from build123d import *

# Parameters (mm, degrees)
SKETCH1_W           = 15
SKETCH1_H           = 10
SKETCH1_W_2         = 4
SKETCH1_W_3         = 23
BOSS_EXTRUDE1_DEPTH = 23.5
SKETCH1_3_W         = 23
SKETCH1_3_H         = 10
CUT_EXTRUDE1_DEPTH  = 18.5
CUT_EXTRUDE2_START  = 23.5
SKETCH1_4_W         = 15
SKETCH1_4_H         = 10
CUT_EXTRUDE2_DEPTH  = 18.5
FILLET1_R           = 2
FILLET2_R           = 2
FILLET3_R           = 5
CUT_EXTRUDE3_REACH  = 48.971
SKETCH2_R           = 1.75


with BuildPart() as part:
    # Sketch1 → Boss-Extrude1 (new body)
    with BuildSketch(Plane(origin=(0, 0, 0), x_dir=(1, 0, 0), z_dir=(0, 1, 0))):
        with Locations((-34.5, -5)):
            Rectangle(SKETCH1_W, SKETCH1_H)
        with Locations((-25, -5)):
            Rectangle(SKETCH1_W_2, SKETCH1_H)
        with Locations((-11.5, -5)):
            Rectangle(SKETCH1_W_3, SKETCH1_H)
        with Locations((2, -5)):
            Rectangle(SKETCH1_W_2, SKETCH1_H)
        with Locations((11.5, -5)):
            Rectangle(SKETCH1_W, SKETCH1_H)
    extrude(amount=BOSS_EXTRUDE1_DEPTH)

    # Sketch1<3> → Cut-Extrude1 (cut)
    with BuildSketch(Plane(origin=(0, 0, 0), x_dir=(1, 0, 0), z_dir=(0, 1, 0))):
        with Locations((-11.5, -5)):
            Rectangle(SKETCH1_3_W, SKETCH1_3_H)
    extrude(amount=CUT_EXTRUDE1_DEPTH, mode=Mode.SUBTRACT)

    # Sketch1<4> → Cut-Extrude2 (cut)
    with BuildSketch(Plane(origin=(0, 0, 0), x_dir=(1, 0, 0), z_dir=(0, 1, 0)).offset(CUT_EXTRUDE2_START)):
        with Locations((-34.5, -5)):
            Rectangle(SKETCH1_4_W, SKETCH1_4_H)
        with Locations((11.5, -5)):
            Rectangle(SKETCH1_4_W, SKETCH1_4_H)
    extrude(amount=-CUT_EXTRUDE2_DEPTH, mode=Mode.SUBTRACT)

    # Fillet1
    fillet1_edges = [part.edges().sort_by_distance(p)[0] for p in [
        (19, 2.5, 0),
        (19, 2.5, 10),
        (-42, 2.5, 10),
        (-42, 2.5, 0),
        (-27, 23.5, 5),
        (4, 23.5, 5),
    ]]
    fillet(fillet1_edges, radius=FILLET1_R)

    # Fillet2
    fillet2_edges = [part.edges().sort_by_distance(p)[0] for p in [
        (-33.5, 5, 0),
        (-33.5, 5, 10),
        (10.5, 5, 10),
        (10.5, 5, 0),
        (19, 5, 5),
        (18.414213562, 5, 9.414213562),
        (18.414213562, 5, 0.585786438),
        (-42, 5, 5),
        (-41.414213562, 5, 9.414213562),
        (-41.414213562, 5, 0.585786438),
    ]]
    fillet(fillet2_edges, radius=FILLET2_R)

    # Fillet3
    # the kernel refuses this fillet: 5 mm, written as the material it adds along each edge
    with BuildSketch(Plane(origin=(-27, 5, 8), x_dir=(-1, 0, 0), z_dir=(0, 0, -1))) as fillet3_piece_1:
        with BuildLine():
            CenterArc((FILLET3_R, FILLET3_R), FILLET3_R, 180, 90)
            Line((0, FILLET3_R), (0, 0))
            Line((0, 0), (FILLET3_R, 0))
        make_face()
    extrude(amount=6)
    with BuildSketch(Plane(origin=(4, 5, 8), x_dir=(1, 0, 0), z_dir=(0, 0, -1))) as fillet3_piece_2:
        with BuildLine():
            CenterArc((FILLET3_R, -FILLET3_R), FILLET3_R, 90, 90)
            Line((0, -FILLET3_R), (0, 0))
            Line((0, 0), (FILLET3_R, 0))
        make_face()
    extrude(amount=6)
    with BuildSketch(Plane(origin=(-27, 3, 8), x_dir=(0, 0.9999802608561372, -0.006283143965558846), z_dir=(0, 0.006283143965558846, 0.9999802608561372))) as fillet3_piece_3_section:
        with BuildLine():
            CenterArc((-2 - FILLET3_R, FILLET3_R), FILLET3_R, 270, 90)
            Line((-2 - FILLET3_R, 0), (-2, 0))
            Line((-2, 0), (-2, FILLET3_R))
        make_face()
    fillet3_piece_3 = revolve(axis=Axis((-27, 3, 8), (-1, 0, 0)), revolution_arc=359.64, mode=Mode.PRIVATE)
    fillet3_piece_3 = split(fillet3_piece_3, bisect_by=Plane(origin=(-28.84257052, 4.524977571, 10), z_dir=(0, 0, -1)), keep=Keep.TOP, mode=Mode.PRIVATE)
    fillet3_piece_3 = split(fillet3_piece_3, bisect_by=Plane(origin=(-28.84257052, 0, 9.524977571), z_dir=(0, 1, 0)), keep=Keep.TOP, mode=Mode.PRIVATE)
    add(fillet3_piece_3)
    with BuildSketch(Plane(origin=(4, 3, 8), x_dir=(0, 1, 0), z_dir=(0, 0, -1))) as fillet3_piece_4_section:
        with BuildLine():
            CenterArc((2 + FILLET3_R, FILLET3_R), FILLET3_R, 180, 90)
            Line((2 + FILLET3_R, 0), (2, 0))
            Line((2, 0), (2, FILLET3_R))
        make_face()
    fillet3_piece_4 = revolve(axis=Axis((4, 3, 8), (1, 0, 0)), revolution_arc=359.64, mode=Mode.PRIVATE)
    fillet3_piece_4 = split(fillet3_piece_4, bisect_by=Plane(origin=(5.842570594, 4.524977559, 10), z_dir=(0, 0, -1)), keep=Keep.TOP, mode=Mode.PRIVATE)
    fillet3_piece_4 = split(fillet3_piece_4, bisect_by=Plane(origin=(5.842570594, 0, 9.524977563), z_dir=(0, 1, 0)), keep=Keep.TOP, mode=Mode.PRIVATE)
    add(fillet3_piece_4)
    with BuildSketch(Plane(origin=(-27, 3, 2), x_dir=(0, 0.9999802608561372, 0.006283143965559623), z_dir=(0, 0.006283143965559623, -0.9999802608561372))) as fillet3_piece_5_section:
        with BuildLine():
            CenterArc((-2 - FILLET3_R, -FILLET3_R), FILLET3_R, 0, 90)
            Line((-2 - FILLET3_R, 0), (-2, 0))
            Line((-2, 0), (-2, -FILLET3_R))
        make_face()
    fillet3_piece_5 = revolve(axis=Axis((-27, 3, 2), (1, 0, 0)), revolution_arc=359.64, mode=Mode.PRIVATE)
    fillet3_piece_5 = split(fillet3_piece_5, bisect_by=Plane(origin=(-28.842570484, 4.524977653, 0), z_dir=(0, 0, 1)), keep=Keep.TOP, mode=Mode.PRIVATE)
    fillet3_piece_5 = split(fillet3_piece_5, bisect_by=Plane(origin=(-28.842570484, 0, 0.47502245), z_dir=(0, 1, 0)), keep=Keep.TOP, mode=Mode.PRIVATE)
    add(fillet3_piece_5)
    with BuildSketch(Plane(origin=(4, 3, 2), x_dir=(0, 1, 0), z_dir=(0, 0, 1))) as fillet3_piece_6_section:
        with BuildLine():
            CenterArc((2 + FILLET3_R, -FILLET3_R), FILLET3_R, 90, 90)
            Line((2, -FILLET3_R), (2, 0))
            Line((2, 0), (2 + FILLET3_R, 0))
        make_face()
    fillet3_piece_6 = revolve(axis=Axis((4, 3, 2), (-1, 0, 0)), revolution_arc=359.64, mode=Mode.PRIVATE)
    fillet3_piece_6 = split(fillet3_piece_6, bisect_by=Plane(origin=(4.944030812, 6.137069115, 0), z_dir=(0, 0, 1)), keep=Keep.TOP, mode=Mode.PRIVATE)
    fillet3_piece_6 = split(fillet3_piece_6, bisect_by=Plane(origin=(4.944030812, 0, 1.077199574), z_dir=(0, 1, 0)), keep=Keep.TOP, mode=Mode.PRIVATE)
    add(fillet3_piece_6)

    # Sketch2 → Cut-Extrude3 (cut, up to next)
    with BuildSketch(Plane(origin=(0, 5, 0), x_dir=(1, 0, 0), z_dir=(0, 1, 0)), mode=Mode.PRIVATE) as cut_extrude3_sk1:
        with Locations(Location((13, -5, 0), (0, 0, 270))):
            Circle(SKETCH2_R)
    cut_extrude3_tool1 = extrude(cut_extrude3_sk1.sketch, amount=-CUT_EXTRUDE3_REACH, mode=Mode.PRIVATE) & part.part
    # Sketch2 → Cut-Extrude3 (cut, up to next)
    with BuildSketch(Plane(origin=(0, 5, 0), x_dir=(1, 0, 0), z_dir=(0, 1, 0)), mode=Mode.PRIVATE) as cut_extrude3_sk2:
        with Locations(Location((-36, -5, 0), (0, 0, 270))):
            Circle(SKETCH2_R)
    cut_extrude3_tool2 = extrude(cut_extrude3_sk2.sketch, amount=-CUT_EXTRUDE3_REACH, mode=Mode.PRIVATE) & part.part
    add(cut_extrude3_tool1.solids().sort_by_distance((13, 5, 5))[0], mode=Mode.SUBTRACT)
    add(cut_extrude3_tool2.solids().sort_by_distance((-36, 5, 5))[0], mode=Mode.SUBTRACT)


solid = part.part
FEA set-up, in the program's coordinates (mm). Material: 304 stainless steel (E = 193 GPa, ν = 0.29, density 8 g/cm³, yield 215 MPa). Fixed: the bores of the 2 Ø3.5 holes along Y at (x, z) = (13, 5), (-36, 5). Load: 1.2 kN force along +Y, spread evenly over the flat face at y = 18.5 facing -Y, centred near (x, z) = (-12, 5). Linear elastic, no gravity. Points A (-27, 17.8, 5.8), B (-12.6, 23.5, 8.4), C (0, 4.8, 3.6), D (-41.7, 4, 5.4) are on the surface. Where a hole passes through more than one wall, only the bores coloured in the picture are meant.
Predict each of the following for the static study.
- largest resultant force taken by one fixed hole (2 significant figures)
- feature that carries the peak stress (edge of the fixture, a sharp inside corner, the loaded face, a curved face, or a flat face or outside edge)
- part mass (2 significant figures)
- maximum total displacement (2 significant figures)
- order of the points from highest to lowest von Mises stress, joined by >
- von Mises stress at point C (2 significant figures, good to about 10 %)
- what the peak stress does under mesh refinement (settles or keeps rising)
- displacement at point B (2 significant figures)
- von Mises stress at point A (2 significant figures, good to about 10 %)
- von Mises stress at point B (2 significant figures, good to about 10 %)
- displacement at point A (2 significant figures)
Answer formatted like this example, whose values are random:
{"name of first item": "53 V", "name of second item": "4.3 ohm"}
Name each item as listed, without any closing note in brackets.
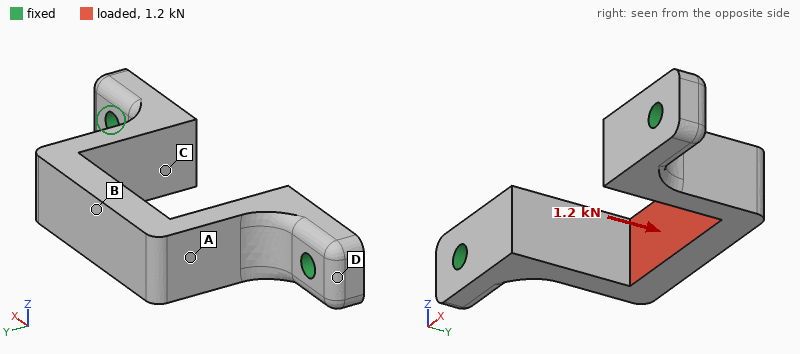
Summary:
{"largest resultant force taken by one fixed hole": "670 N", "feature that carries the peak stress": "edge of the fixture", "part mass": "36 g", "maximum total displacement": "13 µm", "order of the points from highest to lowest von Mises stress, joined by >": "B > A > C > D", "von Mises stress at point C": "17 MPa", "what the peak stress does under mesh refinement": "keeps rising", "displacement at point B": "12 µm", "von Mises stress at point A": "33 MPa", "von Mises stress at point B": "55 MPa", "displacement at point A": "5.3 µm"}
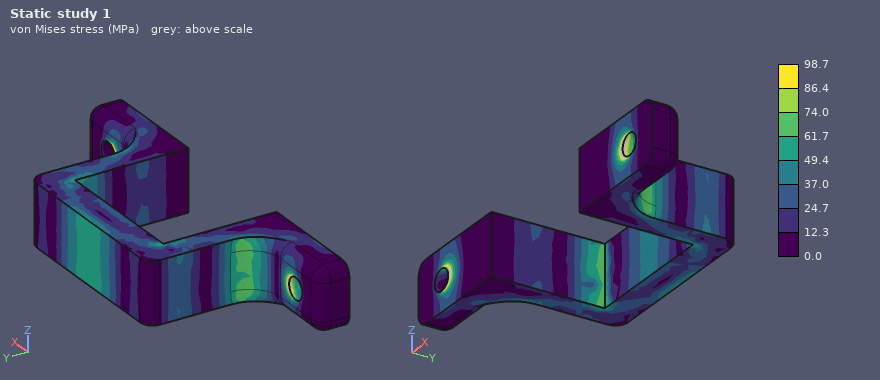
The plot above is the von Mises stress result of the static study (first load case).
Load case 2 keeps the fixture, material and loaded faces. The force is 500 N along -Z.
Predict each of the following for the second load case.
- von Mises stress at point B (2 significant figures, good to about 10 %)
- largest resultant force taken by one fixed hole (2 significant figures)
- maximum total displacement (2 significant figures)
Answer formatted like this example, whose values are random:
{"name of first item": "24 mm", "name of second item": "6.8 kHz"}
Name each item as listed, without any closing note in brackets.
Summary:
{"von Mises stress at point B": "17 MPa", "largest resultant force taken by one fixed hole": "250 N", "maximum total displacement": "38 µm"}
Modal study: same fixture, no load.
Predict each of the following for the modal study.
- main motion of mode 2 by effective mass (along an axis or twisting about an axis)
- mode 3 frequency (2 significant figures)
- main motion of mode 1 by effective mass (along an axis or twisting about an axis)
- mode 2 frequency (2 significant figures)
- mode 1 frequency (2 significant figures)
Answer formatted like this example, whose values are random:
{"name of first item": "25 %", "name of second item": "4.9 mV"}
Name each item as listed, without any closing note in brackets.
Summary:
{"main motion of mode 2 by effective mass": "along X", "mode 3 frequency": "9800 Hz", "main motion of mode 1 by effective mass": "along Z", "mode 2 frequency": "7500 Hz", "mode 1 frequency": "4700 Hz"}
